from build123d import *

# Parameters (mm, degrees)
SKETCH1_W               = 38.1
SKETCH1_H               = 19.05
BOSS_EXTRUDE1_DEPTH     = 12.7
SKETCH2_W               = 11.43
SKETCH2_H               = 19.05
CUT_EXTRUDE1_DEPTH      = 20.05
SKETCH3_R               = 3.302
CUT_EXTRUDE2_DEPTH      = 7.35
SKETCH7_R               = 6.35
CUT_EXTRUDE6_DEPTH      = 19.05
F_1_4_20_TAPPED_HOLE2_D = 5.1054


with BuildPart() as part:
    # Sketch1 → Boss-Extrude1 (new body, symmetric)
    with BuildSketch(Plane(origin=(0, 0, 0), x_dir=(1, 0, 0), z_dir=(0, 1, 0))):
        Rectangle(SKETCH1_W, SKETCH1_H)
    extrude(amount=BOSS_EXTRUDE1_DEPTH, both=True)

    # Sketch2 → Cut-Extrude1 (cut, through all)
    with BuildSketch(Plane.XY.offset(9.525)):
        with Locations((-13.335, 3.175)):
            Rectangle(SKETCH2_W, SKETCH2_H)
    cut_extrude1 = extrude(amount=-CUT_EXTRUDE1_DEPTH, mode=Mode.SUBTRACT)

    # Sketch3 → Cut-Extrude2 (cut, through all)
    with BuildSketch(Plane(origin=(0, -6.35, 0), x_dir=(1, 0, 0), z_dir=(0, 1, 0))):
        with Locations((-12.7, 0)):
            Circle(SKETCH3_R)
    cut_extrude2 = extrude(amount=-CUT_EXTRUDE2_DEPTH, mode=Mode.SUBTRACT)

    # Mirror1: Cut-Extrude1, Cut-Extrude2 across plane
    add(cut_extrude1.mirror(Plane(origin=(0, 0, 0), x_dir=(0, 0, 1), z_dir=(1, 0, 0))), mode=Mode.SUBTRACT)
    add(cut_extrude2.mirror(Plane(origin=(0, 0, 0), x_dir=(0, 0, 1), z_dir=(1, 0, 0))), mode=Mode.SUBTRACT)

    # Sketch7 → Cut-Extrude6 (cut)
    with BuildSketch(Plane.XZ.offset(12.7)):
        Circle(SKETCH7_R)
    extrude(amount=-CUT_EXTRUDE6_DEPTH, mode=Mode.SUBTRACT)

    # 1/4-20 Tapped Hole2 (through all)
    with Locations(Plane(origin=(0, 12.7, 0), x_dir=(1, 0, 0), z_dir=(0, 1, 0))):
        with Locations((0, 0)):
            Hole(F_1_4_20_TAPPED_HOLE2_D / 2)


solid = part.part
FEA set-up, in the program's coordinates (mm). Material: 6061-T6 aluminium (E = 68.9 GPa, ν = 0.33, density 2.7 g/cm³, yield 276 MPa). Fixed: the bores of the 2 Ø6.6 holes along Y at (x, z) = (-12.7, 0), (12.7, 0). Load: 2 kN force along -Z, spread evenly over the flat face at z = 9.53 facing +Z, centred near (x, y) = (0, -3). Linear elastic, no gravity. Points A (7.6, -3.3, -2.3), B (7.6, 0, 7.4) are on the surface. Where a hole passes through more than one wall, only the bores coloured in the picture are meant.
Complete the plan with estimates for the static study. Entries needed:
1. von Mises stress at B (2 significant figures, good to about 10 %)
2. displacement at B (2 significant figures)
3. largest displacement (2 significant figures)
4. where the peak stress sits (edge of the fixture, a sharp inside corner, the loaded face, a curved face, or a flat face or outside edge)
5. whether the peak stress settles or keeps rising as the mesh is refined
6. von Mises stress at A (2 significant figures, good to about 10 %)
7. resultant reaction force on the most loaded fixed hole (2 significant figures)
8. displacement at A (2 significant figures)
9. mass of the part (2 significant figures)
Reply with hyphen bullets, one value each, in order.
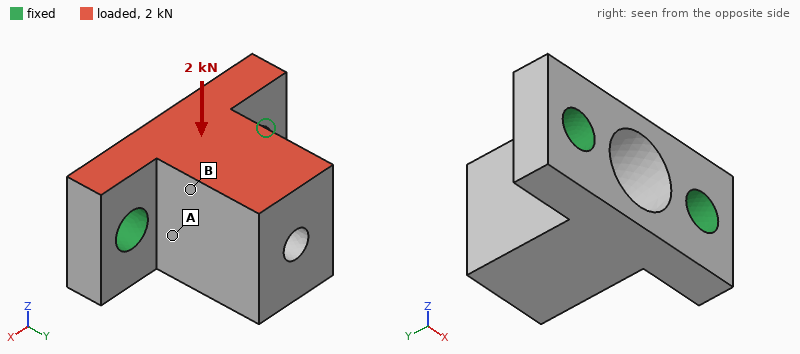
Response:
- 14 MPa
- 16 µm
- 32 µm
- edge of the fixture
- keeps rising
- 32 MPa
- 1.0 kN
- 8.6 µm
- 19 g
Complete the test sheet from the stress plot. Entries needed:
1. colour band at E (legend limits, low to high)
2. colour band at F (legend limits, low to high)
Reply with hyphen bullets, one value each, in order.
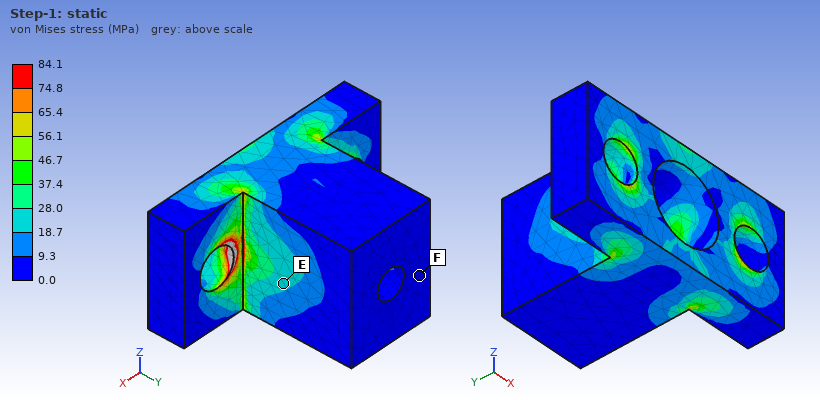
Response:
- 18.7 to 28.0 MPa
- 0.0 to 9.3 MPa
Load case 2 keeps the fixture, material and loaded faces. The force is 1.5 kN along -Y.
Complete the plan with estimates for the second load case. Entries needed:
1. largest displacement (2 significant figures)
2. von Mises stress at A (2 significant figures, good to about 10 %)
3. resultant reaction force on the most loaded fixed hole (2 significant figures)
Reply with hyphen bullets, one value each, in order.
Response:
- 24 µm
- 13 MPa
- 760 N
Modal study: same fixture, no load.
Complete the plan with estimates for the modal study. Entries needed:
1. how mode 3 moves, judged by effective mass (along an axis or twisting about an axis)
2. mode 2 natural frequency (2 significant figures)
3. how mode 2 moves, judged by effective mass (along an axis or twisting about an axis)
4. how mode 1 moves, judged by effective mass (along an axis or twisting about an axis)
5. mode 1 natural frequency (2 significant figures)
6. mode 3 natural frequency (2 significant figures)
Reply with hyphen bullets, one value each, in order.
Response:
- along Y
- 15 kHz
- along X
- along Z
- 10 kHz
- 27 kHz
